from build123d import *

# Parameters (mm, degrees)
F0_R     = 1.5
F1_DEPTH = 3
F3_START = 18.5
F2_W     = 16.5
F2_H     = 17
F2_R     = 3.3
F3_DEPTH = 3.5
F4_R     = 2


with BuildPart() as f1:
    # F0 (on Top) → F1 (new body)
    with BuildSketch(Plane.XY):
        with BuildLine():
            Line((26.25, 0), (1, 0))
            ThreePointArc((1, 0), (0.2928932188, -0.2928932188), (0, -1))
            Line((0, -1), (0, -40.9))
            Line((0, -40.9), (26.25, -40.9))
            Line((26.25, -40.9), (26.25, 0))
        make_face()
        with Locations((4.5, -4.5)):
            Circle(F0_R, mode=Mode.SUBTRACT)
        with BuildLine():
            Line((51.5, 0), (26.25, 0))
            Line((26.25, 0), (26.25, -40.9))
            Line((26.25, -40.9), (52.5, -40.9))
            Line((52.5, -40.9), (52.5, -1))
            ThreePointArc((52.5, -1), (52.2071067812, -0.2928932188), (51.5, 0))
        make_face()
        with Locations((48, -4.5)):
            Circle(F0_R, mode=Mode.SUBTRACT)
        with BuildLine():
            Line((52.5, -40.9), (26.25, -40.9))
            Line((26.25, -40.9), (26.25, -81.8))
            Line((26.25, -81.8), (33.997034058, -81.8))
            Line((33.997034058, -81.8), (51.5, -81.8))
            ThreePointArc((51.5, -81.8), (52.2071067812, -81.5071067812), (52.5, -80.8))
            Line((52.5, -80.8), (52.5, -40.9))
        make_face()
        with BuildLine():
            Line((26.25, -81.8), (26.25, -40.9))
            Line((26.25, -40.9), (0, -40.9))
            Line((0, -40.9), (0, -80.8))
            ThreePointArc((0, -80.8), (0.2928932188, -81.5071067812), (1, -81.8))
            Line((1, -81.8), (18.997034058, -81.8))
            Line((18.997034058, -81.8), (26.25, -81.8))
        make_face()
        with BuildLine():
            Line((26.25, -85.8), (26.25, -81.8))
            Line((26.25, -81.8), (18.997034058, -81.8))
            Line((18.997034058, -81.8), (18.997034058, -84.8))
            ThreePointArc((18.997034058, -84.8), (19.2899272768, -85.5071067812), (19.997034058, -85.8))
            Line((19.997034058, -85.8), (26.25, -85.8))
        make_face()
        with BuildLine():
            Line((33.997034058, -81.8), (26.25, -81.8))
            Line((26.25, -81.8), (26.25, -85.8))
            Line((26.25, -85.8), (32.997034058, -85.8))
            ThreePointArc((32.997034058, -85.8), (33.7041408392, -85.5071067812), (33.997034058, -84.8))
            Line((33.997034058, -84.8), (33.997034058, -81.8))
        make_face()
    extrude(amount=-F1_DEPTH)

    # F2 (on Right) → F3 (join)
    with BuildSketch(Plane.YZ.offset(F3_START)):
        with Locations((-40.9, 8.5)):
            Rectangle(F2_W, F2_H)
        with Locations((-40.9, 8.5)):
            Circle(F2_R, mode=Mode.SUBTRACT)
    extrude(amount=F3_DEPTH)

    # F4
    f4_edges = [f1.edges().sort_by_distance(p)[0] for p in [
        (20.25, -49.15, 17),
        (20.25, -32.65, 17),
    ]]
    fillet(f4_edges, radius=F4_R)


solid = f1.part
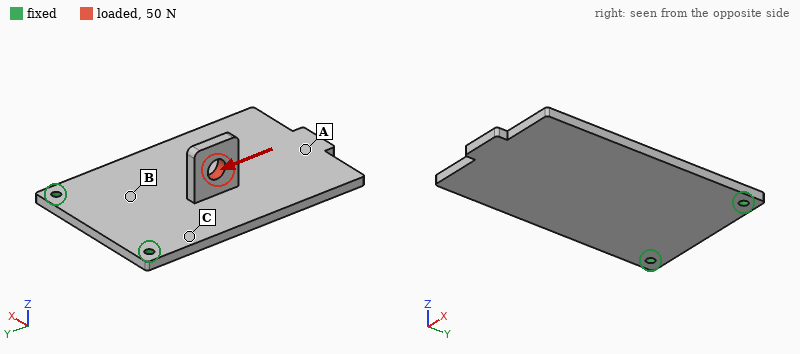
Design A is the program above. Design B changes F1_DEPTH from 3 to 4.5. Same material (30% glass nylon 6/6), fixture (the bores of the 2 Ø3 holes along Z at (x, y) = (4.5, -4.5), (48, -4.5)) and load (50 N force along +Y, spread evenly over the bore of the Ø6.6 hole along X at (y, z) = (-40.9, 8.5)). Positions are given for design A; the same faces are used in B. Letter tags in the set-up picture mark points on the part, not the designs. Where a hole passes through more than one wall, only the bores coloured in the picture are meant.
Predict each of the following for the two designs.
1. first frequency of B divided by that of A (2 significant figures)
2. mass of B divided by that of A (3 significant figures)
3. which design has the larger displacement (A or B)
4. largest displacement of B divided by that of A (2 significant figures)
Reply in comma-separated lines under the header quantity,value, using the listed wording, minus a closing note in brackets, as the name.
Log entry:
quantity,value
first frequency of B divided by that of A,1.5
mass of B divided by that of A,1.47
which design has the larger displacement,A
largest displacement of B divided by that of A,0.34
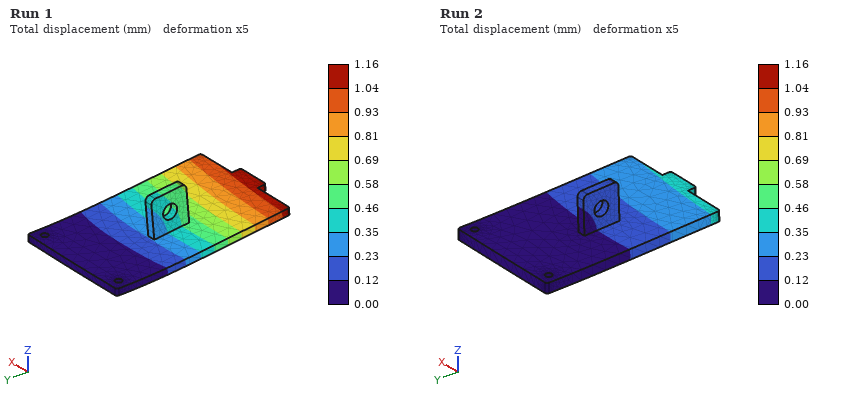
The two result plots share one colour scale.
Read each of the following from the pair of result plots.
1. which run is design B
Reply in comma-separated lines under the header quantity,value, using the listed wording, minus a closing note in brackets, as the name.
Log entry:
quantity,value
which run is design B,Run 2
